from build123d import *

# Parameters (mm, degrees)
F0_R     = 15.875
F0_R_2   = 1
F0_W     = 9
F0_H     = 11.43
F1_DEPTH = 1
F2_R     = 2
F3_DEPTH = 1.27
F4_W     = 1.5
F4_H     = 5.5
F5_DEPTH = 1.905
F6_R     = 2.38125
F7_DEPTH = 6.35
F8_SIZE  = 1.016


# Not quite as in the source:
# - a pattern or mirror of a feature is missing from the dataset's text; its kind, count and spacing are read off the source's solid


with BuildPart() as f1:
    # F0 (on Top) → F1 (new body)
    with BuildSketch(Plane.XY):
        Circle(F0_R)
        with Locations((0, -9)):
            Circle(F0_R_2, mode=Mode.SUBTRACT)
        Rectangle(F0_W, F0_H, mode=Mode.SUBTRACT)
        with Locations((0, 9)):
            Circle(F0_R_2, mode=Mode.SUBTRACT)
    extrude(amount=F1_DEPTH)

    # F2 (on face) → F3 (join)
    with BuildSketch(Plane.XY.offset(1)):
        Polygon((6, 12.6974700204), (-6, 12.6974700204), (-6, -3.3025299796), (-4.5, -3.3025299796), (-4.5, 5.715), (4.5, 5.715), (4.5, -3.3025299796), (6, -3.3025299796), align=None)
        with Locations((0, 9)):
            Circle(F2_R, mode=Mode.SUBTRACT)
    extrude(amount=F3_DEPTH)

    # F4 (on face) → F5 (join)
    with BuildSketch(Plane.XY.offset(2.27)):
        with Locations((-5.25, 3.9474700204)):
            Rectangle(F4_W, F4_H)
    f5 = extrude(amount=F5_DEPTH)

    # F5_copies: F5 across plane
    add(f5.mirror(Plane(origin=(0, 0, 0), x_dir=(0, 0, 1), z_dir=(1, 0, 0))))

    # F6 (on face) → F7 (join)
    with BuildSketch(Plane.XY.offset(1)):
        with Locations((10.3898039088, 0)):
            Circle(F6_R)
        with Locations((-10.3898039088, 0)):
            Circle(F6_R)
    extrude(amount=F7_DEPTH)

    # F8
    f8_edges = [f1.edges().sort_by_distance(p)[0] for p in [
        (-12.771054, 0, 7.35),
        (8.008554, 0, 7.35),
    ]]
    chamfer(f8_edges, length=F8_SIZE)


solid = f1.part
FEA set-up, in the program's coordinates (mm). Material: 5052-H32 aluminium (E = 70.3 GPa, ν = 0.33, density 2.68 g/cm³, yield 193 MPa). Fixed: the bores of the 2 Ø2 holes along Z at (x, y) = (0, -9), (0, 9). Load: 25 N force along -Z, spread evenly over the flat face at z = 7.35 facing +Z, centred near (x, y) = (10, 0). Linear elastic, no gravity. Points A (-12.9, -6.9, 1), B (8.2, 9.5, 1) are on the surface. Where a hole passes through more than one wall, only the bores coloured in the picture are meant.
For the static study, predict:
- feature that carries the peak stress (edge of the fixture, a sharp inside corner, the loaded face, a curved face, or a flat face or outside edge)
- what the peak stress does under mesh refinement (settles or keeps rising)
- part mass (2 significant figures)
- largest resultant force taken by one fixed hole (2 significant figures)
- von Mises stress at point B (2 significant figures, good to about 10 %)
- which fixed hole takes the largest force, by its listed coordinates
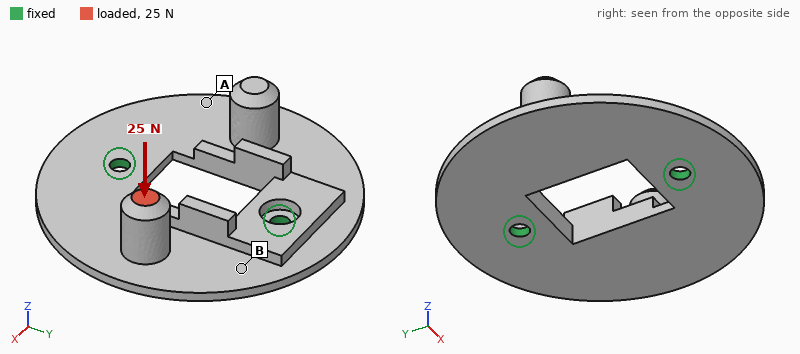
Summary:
edge of the fixture
keeps rising
2.8 g
15 N
23 MPa
(0, 9)
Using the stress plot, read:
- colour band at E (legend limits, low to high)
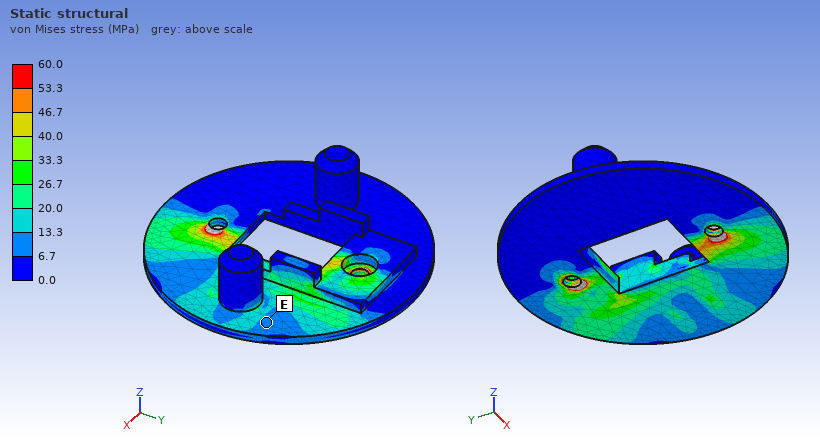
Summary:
6.7 to 13.3 MPa
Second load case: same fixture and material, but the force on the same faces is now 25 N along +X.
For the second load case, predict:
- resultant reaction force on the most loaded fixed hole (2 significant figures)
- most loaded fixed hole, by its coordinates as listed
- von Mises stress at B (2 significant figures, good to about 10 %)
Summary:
15 N
(0, 9)
33 MPa
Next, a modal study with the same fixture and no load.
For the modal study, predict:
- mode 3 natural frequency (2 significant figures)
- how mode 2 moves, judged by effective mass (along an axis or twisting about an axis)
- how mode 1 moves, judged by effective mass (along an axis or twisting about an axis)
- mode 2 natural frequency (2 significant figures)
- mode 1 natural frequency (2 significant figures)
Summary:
8800 Hz
along Z
twisting about Y
3900 Hz
3400 Hz
